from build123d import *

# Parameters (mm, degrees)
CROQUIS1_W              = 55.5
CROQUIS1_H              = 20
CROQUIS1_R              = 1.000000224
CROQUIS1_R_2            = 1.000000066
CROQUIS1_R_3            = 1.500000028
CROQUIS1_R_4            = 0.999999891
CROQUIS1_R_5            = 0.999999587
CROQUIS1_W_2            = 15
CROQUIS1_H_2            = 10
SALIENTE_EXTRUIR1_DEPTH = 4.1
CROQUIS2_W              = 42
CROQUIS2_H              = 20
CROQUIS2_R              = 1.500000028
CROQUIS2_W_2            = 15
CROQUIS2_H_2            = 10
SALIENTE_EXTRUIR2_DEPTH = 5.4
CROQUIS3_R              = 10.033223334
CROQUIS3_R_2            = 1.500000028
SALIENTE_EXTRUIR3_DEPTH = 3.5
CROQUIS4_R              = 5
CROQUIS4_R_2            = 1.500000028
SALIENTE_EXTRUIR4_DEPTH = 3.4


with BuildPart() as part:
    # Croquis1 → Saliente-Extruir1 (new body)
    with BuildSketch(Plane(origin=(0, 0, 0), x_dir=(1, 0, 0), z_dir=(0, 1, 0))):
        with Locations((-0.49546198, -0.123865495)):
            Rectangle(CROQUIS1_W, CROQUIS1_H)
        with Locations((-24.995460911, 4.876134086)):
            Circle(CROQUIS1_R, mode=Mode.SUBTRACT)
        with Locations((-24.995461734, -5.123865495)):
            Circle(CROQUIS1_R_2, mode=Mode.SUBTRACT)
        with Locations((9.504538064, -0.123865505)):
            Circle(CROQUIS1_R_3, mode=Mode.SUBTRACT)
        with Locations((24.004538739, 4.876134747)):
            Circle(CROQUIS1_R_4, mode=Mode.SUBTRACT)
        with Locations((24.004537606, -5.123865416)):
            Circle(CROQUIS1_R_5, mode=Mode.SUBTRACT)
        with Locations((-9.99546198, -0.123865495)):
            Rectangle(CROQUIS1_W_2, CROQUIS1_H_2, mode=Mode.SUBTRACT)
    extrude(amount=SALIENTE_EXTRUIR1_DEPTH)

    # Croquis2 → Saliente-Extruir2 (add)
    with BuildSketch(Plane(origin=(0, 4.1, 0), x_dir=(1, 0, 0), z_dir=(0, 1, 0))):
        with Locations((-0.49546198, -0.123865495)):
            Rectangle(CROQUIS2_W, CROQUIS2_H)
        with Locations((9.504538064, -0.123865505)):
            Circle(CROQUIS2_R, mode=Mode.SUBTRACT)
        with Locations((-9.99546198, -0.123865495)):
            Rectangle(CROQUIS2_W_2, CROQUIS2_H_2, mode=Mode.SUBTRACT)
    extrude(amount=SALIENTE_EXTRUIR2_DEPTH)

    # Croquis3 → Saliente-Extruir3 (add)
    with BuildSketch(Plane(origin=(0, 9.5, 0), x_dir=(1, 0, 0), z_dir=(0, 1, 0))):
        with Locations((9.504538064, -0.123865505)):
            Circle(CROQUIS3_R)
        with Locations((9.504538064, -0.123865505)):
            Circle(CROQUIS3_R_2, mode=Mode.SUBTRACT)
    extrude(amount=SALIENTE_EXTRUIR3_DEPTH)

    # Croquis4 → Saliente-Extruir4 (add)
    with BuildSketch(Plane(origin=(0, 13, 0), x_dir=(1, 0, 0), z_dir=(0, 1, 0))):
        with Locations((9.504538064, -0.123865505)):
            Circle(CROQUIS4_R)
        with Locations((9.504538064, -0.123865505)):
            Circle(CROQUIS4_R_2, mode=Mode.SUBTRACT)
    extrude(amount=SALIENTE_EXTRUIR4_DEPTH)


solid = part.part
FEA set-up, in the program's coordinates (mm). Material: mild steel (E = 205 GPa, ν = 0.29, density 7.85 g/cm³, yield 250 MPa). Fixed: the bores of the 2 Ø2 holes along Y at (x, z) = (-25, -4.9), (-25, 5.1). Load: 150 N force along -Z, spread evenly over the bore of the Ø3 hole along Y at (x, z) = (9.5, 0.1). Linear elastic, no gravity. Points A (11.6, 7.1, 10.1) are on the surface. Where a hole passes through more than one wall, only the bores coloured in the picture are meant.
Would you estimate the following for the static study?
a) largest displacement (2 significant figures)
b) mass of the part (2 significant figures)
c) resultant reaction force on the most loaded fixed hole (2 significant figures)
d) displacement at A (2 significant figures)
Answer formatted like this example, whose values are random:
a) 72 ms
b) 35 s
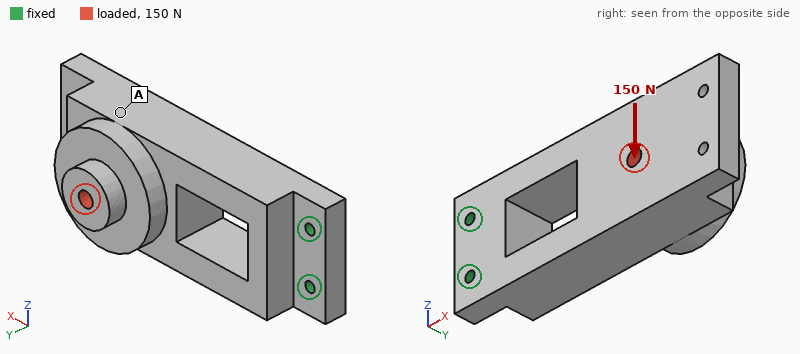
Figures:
a) 11 µm
b) 70 g
c) 460 N
d) 8.6 µm
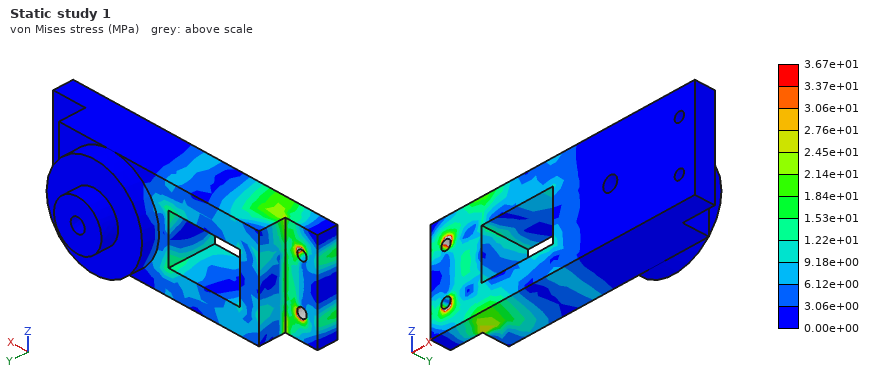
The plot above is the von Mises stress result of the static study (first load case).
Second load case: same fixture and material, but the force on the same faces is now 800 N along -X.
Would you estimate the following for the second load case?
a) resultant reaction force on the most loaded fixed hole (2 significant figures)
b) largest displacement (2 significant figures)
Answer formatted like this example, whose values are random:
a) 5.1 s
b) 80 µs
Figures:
a) 400 N
b) 81 µm
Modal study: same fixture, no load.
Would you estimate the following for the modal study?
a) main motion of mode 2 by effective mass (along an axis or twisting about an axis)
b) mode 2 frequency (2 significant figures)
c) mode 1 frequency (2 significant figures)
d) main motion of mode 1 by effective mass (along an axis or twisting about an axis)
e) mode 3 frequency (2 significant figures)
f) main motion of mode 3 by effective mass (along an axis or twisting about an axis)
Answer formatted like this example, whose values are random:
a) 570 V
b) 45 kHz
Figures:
a) along Z
b) 2900 Hz
c) 1100 Hz
d) along Y
e) 5900 Hz
f) twisting about X
